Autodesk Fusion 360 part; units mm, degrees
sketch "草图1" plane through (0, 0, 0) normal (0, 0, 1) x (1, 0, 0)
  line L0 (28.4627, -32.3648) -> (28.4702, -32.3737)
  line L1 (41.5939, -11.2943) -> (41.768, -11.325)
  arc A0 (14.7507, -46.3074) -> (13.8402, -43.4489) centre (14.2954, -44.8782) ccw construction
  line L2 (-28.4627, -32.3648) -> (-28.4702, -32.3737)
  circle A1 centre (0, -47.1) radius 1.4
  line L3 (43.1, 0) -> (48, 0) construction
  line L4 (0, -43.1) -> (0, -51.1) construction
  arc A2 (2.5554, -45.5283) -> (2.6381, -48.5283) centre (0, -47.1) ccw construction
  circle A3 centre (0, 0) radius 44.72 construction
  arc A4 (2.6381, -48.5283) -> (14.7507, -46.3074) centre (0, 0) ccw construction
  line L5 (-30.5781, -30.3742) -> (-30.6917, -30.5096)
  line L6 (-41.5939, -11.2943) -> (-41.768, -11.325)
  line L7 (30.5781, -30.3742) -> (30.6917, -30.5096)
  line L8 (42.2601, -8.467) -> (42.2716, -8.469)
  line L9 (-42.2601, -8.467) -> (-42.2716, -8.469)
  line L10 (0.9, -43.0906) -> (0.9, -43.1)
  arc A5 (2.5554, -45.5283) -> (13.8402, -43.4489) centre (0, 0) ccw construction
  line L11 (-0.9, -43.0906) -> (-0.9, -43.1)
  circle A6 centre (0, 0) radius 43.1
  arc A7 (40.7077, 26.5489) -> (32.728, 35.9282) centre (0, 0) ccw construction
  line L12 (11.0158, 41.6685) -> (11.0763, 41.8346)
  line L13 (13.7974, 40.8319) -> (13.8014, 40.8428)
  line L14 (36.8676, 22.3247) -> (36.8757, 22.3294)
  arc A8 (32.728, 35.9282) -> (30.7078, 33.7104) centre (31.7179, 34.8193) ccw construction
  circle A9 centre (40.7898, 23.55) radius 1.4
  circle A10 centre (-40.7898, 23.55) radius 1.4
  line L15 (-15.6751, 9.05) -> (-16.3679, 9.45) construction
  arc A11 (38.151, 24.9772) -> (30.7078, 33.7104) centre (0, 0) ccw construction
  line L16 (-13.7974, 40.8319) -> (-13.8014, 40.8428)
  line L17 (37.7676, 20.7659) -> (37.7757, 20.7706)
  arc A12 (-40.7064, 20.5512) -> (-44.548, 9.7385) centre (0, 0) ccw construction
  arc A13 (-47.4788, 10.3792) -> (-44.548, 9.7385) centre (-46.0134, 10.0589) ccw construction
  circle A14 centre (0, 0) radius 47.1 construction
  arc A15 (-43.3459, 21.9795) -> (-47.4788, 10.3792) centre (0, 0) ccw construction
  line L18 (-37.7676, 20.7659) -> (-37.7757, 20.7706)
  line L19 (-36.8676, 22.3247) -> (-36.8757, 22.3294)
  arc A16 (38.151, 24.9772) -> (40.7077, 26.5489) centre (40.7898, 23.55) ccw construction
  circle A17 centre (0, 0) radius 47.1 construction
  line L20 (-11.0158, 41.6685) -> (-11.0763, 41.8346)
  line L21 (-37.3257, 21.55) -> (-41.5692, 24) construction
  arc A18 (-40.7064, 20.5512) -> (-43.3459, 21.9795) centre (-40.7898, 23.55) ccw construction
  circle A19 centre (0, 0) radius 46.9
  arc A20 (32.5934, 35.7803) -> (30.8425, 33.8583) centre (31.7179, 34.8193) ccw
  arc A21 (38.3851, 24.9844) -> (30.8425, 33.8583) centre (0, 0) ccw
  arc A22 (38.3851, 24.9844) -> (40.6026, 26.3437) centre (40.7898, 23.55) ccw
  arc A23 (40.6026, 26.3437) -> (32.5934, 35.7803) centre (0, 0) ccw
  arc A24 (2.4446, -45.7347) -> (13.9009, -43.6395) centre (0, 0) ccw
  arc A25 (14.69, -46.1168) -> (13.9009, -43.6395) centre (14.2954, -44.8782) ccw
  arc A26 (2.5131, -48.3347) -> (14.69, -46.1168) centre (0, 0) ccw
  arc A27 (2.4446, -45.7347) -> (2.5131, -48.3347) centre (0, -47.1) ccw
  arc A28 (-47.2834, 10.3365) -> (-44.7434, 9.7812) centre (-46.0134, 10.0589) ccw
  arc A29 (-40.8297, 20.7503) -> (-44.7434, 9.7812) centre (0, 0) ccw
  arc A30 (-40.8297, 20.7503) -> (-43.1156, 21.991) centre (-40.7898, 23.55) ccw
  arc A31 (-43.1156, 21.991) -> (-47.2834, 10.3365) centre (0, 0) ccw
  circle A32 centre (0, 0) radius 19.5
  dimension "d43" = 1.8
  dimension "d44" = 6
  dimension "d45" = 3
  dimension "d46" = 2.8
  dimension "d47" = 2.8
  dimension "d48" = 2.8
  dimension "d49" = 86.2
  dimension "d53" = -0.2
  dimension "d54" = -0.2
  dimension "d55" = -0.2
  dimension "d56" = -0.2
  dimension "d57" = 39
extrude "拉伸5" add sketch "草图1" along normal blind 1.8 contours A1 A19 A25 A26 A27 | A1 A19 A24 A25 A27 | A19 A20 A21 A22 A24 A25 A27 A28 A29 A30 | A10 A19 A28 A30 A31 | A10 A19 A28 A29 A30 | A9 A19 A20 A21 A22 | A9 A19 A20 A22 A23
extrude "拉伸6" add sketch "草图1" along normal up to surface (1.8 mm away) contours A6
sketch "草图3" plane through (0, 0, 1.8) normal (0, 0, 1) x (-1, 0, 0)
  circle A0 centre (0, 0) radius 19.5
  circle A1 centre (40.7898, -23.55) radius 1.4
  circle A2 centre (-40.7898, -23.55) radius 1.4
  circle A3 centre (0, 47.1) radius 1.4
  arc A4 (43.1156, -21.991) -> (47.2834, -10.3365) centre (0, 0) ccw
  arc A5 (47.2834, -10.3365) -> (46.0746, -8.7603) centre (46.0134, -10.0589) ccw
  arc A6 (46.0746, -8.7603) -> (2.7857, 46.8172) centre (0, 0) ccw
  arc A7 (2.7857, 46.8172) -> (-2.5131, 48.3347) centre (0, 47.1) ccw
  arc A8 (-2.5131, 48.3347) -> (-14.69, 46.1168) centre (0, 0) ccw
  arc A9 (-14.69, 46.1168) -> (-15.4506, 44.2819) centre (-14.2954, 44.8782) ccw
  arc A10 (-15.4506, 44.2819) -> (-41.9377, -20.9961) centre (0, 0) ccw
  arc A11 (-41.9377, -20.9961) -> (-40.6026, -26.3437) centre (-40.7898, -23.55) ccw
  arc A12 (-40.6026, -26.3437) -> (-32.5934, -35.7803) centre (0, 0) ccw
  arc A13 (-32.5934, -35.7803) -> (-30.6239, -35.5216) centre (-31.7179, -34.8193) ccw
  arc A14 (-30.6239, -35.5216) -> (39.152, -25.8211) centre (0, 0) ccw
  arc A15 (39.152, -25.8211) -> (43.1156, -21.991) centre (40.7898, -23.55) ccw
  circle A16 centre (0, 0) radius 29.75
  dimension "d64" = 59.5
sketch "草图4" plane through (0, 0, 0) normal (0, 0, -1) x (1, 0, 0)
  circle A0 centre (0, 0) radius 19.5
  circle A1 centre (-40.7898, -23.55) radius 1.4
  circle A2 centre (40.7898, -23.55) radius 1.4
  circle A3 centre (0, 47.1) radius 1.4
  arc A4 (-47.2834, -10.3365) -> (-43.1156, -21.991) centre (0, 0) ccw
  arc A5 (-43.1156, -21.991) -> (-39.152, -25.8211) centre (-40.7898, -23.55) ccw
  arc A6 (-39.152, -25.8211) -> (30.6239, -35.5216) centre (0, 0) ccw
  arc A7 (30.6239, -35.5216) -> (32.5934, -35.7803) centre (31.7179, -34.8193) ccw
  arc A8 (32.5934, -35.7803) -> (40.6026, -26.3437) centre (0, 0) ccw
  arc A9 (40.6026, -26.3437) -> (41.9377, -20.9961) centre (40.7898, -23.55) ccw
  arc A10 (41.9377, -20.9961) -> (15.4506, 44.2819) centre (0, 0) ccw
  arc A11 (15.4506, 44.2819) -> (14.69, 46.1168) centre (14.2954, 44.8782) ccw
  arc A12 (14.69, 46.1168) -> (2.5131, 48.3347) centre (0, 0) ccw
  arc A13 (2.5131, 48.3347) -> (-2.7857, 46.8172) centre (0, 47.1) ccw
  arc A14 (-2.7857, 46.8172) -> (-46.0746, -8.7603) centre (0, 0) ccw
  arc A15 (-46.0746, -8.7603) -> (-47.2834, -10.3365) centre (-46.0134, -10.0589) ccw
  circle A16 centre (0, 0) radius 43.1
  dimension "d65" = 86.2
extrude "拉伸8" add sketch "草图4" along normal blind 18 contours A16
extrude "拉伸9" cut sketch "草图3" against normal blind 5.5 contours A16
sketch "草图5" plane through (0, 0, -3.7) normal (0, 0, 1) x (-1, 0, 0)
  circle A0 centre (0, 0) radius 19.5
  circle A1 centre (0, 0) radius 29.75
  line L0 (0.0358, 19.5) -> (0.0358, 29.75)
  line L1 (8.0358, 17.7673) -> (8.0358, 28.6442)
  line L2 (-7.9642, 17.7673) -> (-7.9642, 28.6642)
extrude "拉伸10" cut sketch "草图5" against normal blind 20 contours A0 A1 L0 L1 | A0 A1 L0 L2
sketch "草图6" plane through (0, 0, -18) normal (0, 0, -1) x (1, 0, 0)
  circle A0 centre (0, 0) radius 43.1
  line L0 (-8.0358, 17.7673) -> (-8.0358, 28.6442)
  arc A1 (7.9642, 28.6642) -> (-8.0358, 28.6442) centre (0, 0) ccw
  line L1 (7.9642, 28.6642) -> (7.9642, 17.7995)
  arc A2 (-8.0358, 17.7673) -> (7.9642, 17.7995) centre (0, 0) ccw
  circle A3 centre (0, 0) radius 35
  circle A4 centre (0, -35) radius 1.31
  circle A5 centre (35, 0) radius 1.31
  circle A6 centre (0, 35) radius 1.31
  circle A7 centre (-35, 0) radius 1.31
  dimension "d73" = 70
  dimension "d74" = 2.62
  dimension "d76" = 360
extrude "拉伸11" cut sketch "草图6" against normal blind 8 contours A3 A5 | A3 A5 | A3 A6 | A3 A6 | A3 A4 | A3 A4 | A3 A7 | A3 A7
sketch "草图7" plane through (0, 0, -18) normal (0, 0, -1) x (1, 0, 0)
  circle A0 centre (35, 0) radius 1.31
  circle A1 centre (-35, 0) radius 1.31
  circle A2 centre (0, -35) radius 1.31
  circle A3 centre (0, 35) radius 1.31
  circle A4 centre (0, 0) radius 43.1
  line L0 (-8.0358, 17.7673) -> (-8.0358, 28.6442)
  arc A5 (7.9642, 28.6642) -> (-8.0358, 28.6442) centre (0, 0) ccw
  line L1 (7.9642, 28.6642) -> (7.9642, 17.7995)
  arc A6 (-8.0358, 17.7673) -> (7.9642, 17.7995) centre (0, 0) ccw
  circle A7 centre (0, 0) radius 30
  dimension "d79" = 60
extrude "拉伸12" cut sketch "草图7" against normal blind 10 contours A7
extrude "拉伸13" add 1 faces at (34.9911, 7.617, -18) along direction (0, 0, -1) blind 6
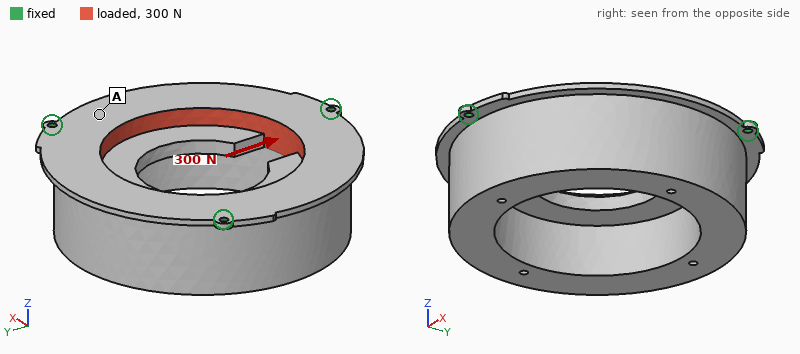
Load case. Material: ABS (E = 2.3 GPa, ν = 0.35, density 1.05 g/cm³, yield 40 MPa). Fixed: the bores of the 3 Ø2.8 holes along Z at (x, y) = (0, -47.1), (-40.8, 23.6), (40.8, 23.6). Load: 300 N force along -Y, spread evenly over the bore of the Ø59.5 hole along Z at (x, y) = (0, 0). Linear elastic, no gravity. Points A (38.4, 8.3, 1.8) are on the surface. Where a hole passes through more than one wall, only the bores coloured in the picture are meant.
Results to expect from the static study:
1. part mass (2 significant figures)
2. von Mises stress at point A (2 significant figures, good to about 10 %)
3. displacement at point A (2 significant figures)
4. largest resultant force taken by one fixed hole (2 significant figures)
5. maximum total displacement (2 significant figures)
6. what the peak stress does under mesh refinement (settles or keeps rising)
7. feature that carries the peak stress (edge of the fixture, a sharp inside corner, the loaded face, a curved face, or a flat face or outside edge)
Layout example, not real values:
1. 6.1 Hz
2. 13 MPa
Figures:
1. 90 g
2. 0.96 MPa
3. 27 µm
4. 100 N
5. 42 µm
6. keeps rising
7. edge of the fixture
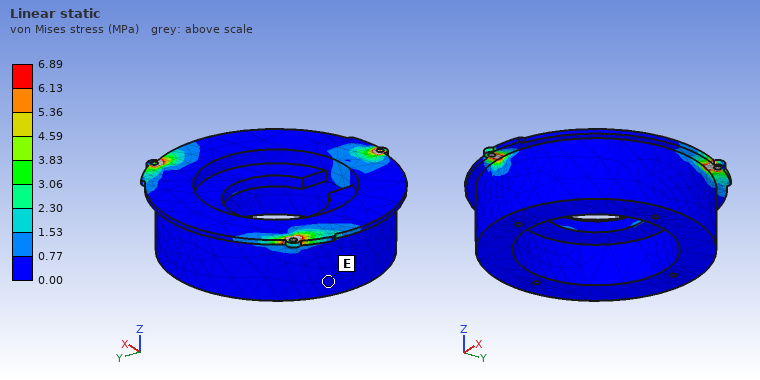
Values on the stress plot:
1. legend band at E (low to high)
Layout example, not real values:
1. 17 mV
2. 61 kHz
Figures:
1. 0.00 to 0.77 MPa
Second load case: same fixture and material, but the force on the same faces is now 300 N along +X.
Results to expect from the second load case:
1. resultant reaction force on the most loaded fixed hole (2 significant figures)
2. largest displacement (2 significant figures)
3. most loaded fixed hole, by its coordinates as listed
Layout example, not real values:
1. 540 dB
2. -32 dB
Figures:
1. 110 N
2. 42 µm
3. (0, -47.1)
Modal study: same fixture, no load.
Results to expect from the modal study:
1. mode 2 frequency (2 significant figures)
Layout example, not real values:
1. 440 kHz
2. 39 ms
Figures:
1. 910 Hz
